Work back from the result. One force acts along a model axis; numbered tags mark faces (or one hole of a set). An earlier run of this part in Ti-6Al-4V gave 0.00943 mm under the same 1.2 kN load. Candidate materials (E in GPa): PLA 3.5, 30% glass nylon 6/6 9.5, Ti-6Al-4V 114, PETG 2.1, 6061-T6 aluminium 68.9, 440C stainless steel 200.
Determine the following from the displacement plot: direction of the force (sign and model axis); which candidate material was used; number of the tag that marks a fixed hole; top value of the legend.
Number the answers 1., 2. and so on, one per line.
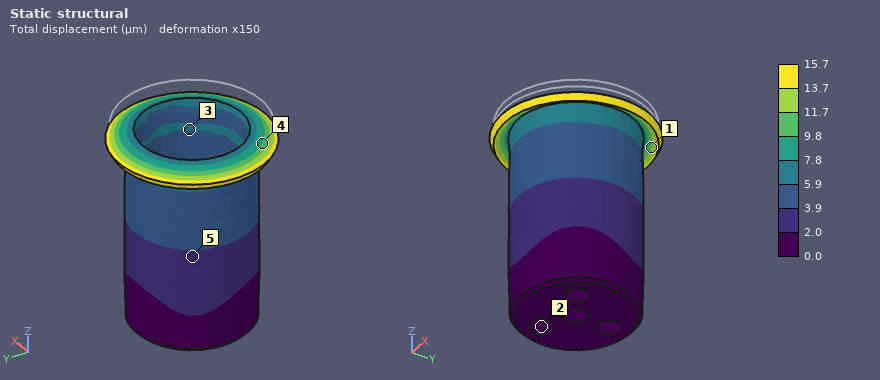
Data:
1. -Z
2. 6061-T6 aluminium
3. 2
4. 15.7 µm
